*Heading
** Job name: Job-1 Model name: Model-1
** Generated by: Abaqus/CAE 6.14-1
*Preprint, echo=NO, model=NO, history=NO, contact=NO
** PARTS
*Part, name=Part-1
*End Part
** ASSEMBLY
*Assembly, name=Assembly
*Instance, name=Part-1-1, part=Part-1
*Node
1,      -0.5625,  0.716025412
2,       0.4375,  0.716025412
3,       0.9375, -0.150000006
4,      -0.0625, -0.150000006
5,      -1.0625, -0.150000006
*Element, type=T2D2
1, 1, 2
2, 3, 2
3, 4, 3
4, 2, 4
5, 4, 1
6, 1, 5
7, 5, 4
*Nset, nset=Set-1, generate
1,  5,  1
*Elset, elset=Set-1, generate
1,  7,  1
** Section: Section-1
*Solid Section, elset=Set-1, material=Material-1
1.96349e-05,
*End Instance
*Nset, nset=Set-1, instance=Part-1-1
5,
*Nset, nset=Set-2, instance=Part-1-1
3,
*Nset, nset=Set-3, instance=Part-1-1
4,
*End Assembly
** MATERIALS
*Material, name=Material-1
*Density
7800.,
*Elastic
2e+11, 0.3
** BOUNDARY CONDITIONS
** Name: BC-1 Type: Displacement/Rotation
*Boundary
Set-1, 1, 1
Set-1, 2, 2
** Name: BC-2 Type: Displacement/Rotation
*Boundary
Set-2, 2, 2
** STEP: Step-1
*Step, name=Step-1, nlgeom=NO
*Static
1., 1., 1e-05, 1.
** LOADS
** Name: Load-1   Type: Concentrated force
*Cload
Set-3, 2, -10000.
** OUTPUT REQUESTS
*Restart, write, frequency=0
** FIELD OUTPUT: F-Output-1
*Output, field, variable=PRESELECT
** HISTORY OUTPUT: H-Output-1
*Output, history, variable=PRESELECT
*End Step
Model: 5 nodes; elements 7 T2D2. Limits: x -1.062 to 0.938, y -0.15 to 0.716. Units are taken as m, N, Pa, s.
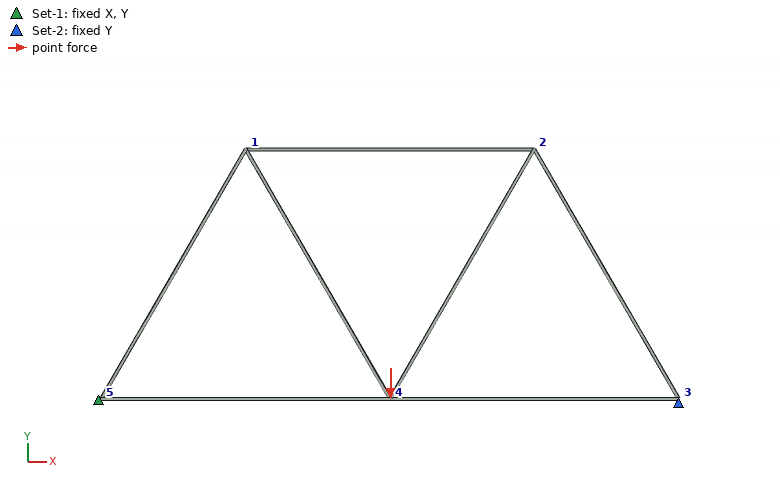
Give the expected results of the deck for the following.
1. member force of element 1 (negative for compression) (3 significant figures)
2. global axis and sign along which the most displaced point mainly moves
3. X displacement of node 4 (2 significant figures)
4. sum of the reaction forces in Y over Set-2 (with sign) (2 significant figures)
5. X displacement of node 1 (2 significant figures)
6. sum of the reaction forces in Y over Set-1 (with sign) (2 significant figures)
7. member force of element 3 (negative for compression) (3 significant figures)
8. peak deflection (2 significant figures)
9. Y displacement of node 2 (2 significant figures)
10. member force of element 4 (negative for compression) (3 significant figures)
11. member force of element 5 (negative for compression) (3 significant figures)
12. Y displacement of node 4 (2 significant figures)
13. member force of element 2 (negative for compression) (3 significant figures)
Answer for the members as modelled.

-5770 N
-Y
7.4e-04 m
5000 N
0.0015 m
5000 N
2890 N
0.0047 m
-0.0025 m
5770 N
5770 N
-0.0047 m
-5770 N
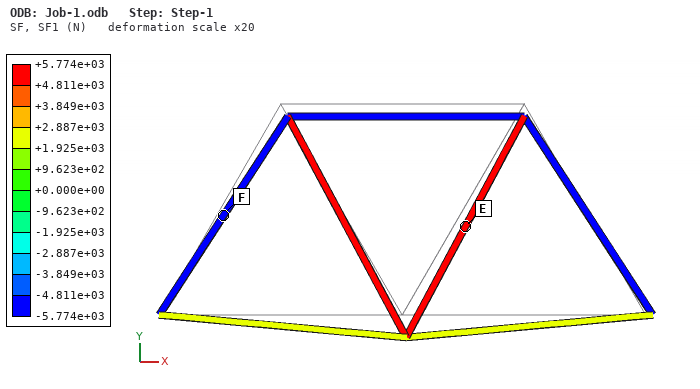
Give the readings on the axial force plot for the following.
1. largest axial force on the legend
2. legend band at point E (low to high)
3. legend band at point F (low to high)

+5.774e+03 N
+4.811e+03 to +5.774e+03 N
-5.774e+03 to -4.811e+03 N
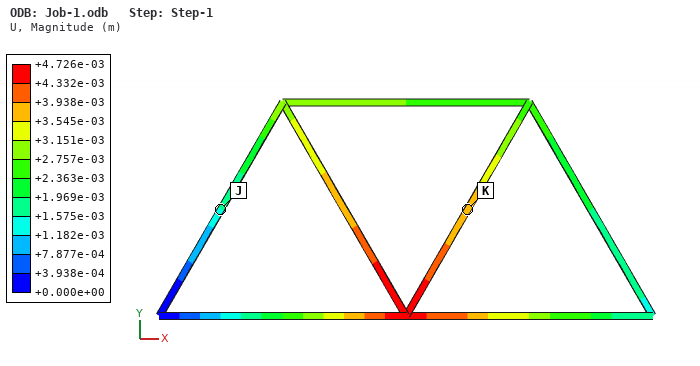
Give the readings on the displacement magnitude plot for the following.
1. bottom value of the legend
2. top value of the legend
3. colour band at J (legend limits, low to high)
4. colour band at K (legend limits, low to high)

+0.000e+00 m
+4.726e-03 m
+1.182e-03 to +1.575e-03 m
+3.545e-03 to +3.938e-03 m
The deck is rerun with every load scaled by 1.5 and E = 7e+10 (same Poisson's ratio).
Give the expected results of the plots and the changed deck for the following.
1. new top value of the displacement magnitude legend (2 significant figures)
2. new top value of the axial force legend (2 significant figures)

0.020 m
8700 N
